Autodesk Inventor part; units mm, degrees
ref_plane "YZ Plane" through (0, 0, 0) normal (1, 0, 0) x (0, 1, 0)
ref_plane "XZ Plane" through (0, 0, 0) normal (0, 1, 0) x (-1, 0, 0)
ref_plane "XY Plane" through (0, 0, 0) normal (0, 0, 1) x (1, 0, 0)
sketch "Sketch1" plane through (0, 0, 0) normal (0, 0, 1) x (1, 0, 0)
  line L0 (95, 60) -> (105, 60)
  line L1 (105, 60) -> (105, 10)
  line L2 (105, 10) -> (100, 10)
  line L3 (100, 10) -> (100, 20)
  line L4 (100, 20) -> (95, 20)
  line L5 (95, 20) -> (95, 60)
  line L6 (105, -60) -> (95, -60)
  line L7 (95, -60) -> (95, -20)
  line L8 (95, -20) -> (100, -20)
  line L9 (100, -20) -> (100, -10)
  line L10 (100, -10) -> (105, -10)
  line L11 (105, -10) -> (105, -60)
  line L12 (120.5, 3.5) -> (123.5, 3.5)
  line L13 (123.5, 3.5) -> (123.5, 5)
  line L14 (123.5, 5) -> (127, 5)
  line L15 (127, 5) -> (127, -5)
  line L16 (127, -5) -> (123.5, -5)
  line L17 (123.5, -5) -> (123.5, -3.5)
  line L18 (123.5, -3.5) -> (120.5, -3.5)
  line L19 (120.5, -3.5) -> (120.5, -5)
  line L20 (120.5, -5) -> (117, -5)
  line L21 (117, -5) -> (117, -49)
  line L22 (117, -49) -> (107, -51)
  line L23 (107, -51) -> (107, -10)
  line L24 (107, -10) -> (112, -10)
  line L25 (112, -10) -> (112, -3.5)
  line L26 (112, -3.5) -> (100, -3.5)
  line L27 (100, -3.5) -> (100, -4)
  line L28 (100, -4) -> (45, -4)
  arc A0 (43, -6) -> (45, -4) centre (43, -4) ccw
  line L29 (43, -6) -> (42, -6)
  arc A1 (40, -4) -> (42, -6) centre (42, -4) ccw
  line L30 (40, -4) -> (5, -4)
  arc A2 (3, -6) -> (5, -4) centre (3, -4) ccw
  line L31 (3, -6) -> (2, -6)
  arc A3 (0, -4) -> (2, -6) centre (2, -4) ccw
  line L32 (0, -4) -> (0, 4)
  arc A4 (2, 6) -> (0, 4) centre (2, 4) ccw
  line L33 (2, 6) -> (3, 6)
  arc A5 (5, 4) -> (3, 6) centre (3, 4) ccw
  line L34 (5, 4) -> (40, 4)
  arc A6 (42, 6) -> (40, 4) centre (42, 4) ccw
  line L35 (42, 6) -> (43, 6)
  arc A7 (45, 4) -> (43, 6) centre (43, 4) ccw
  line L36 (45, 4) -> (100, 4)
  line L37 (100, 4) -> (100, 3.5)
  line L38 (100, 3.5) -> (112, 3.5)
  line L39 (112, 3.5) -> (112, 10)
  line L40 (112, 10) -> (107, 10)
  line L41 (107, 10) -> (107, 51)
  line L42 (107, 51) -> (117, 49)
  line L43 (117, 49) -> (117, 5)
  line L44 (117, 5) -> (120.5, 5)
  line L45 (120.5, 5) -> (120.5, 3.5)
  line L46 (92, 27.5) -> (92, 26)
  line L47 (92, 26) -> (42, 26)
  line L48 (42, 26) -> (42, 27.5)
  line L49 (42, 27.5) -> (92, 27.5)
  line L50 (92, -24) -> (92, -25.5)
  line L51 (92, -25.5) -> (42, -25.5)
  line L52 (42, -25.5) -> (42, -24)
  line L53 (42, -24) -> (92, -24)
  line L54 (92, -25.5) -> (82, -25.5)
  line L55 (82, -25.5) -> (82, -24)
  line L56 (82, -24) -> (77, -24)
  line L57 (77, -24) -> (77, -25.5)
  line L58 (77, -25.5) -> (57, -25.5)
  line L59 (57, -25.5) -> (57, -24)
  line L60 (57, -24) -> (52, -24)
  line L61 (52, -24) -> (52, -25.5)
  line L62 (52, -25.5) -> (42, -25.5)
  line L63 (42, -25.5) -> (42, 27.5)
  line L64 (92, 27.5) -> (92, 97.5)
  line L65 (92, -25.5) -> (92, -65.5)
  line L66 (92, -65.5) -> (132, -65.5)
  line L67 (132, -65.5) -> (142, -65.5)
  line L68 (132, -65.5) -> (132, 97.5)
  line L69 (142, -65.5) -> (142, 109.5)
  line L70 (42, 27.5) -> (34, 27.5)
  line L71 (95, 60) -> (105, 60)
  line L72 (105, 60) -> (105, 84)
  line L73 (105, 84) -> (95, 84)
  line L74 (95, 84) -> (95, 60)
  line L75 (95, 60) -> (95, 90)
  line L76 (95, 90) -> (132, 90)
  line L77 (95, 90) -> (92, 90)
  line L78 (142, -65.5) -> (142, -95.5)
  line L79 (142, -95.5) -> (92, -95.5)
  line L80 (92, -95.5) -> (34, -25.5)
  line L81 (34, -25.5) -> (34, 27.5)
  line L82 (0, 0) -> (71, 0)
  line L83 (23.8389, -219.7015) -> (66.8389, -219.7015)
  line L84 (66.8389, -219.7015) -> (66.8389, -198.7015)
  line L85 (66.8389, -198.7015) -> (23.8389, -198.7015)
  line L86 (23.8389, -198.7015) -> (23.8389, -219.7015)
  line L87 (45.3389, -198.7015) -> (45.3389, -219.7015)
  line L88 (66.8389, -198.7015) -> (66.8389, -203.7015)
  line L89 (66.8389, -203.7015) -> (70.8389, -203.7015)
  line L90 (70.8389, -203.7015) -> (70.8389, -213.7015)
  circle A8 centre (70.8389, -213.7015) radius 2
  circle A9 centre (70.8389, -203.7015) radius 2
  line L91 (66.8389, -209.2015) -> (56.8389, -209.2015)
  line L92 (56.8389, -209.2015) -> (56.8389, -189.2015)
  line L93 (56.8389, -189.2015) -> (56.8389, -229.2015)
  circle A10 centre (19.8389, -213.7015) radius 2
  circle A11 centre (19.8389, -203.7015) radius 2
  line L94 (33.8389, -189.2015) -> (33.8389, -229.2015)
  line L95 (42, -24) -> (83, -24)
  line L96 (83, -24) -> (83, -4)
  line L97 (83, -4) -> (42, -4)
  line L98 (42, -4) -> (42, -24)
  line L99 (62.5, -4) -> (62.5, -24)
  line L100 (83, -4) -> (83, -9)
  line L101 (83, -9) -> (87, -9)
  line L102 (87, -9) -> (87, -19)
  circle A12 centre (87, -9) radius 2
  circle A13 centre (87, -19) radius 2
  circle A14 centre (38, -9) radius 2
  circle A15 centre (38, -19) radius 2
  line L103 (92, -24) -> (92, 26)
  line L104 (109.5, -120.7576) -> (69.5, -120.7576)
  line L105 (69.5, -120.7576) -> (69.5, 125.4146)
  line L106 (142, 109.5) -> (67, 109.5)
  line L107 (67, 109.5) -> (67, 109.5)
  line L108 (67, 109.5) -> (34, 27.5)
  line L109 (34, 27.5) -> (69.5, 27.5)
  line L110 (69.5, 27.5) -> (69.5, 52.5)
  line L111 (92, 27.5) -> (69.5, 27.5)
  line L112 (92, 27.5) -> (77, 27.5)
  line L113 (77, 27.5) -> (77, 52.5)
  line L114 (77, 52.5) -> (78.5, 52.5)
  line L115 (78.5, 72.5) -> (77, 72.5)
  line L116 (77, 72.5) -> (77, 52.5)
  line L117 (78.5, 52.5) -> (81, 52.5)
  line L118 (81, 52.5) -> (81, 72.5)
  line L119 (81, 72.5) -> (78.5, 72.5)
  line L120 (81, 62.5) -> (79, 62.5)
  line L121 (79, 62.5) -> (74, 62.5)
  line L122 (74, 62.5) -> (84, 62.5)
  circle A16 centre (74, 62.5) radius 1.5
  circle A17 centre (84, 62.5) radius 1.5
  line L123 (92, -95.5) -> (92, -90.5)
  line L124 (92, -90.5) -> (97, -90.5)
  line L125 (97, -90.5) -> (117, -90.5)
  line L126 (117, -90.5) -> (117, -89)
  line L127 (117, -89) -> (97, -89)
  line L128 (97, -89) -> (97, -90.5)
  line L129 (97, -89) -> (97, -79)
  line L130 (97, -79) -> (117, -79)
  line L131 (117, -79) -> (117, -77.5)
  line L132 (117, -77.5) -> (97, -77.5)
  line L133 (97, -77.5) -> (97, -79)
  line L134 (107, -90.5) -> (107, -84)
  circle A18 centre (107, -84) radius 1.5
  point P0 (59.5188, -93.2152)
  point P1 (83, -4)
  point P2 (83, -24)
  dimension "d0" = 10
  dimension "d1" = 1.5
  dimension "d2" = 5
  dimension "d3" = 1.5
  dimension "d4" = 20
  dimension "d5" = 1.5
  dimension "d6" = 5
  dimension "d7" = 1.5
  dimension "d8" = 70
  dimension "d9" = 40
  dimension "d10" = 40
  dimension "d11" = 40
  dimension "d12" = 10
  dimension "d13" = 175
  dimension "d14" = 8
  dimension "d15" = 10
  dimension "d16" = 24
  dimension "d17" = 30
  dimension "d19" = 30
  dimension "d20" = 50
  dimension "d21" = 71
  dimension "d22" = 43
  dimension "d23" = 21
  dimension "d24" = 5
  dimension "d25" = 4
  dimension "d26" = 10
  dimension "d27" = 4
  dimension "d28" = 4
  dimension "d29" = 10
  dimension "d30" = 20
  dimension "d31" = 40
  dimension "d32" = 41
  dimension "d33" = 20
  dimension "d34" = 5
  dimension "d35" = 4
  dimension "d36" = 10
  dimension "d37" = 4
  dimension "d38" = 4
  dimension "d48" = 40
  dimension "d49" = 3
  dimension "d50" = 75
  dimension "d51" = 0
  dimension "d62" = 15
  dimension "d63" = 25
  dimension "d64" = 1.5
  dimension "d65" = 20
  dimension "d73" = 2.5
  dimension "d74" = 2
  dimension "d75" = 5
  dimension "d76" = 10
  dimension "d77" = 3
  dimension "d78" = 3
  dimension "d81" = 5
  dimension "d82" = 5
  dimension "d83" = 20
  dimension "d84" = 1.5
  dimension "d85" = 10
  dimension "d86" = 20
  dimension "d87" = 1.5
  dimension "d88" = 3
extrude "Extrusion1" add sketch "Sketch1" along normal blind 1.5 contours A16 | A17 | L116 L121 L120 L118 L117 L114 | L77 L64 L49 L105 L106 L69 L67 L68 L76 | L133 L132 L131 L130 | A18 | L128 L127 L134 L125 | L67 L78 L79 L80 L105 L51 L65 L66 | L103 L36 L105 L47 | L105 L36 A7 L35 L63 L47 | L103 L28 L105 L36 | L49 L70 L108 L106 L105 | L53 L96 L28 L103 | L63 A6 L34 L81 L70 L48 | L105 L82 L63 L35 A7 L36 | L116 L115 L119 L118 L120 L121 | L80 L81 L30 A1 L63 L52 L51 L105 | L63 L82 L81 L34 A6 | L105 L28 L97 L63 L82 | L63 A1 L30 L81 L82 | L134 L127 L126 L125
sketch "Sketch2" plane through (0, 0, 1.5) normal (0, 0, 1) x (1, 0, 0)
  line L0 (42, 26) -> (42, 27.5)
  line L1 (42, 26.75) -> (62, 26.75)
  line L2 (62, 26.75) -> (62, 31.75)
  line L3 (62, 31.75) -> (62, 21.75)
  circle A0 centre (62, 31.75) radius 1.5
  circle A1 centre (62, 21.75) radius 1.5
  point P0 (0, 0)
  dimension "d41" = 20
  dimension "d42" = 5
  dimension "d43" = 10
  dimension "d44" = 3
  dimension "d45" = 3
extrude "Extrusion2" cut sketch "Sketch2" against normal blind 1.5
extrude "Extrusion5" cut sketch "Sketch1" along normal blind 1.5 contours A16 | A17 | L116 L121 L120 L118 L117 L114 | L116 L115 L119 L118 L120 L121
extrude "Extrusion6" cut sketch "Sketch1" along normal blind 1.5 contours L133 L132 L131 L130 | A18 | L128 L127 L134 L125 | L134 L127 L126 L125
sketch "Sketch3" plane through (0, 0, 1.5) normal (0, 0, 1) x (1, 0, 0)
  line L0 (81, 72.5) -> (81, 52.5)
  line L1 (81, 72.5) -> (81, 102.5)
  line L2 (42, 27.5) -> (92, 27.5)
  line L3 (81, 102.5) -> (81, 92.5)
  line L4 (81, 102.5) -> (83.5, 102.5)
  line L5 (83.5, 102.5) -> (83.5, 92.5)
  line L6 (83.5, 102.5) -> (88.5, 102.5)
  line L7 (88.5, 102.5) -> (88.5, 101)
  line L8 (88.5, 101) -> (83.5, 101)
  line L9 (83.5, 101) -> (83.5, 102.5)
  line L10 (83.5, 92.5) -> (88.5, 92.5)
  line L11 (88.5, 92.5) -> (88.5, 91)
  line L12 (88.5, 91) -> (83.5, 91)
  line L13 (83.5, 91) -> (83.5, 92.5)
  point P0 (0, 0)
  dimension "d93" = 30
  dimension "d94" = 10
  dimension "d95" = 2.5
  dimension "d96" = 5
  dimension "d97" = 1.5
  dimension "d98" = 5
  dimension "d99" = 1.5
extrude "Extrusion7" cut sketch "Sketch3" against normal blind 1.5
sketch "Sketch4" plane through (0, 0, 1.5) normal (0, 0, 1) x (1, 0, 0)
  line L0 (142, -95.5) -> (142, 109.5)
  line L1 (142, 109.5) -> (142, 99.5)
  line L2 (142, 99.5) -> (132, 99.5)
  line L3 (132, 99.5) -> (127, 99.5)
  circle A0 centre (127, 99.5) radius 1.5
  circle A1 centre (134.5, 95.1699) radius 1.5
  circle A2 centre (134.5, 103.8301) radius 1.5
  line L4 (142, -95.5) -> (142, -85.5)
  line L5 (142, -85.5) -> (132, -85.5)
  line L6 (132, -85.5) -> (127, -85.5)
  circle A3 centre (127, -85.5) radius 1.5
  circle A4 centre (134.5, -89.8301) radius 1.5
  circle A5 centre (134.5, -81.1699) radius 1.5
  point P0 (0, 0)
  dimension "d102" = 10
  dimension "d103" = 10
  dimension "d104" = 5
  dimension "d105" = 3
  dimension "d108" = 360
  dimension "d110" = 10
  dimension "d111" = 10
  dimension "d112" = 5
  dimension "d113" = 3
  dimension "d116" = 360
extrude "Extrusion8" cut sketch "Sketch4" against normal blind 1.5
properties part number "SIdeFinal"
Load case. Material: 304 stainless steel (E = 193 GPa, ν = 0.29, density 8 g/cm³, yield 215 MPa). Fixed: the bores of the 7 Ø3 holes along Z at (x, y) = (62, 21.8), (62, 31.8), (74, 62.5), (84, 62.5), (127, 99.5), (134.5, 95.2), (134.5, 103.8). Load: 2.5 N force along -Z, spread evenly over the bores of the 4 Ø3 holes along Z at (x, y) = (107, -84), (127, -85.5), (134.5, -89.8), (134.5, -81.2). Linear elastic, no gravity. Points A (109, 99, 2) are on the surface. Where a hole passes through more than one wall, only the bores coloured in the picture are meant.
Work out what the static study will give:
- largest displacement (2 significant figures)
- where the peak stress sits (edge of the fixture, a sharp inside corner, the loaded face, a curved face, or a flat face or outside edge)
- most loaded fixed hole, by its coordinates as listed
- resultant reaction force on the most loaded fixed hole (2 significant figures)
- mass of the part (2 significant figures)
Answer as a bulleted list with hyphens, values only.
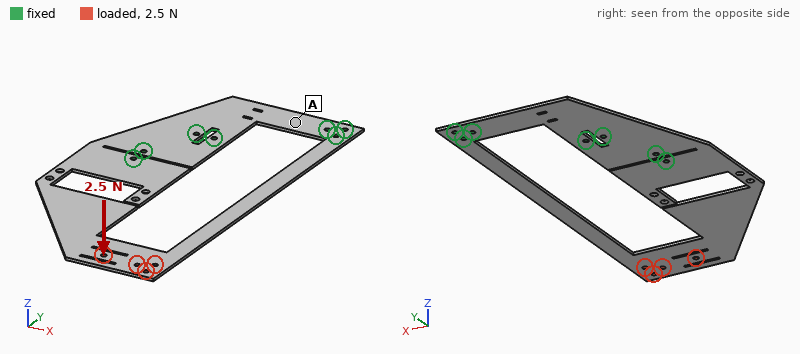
- 2.5 mm
- a curved face
- (134.5, 95.2)
- 6.7 N
- 140 g
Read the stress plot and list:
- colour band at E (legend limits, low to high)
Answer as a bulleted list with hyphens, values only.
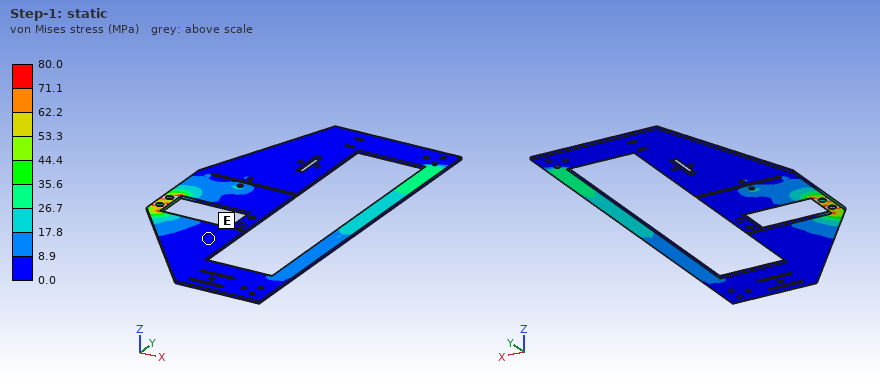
- 0.0 to 8.9 MPa
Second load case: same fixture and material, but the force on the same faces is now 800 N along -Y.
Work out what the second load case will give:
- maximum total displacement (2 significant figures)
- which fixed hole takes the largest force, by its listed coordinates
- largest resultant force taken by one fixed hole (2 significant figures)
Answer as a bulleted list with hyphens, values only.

- 62 µm
- (134.5, 95.2)
- 570 N
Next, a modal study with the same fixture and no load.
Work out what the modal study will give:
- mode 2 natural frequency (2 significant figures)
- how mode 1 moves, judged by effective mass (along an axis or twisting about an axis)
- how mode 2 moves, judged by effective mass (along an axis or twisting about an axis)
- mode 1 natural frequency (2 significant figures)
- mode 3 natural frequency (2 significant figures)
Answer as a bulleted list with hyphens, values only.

- 160 Hz
- along Z
- twisting about Y
- 36 Hz
- 260 Hz
